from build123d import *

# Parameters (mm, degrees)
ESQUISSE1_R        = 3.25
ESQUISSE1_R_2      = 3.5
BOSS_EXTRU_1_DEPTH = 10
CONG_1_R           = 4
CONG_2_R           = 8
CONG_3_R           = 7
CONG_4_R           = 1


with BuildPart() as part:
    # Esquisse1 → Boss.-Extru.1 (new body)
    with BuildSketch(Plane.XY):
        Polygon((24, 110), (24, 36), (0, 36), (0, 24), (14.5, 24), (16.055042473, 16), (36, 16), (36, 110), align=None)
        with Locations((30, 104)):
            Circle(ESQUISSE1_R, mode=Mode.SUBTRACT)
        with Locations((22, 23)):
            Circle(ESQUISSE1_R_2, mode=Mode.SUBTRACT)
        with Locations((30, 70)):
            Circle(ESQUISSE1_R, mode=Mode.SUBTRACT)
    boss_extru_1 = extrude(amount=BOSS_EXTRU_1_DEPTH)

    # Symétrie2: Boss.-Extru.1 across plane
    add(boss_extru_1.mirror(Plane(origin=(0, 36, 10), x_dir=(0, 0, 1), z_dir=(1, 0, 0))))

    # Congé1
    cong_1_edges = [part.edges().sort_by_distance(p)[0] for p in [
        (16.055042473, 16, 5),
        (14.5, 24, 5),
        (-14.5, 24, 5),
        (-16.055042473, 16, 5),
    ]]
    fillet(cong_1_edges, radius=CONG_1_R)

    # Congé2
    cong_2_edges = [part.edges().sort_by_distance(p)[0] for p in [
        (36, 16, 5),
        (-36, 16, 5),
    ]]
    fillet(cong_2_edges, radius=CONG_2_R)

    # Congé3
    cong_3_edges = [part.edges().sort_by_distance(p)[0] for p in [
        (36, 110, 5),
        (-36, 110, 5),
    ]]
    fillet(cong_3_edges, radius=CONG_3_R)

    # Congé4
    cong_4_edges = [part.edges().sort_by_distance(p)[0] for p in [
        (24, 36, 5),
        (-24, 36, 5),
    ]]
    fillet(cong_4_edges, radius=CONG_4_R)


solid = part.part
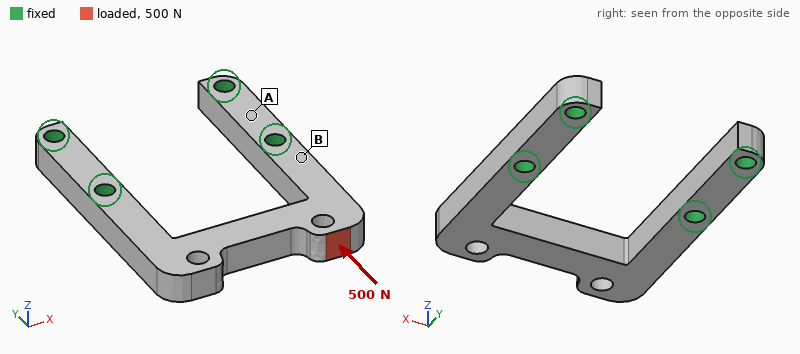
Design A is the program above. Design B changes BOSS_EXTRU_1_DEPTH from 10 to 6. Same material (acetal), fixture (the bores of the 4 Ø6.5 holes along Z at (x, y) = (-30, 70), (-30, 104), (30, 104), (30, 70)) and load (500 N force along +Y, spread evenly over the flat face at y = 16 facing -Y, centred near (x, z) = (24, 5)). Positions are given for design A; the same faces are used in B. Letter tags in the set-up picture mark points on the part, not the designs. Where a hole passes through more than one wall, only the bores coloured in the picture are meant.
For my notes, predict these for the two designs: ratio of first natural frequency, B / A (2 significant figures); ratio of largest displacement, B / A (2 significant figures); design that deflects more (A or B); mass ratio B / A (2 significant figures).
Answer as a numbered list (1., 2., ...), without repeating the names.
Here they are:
1. 0.62
2. 1.7
3. B
4. 0.60
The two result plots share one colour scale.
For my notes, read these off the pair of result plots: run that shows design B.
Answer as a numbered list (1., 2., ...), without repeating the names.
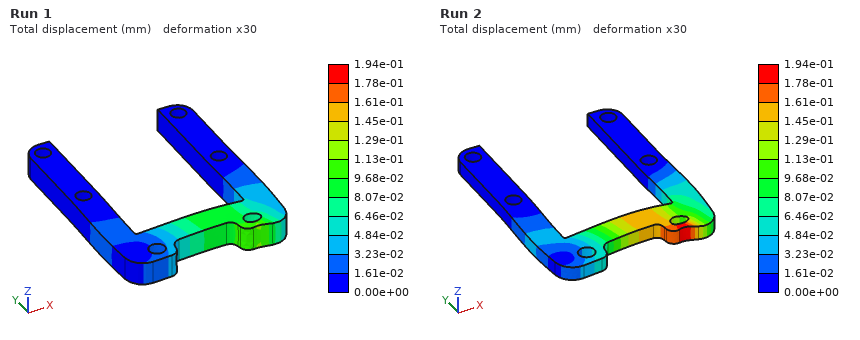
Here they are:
1. Run 2
